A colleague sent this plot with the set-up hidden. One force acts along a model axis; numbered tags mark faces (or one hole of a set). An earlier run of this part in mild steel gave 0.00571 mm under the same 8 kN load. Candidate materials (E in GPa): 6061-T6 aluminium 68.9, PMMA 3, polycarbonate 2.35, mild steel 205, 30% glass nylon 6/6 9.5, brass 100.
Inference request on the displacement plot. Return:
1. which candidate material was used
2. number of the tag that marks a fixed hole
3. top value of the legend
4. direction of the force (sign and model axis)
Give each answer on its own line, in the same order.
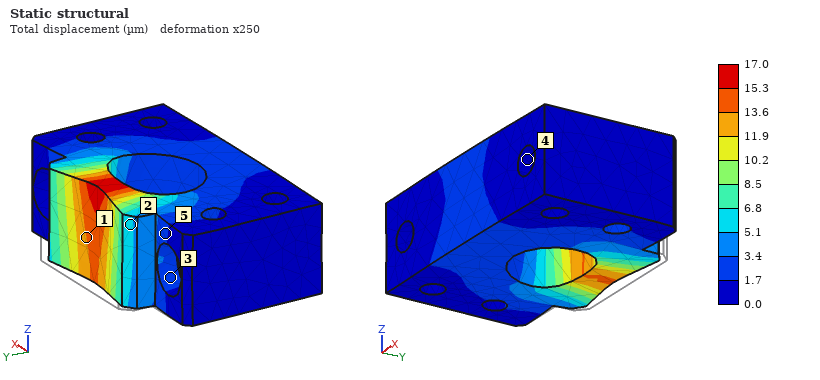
6061-T6 aluminium
4
17.0 µm
-Y
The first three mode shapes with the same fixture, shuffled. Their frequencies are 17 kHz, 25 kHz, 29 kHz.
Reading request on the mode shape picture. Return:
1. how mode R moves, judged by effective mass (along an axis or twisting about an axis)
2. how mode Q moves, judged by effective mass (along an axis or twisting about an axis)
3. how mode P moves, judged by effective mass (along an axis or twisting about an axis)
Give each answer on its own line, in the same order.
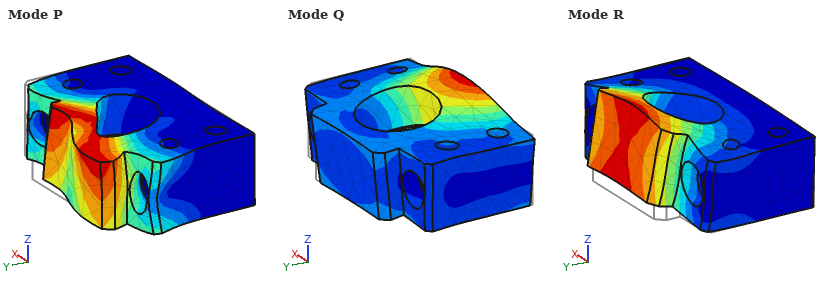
along Z
along Z
along X
